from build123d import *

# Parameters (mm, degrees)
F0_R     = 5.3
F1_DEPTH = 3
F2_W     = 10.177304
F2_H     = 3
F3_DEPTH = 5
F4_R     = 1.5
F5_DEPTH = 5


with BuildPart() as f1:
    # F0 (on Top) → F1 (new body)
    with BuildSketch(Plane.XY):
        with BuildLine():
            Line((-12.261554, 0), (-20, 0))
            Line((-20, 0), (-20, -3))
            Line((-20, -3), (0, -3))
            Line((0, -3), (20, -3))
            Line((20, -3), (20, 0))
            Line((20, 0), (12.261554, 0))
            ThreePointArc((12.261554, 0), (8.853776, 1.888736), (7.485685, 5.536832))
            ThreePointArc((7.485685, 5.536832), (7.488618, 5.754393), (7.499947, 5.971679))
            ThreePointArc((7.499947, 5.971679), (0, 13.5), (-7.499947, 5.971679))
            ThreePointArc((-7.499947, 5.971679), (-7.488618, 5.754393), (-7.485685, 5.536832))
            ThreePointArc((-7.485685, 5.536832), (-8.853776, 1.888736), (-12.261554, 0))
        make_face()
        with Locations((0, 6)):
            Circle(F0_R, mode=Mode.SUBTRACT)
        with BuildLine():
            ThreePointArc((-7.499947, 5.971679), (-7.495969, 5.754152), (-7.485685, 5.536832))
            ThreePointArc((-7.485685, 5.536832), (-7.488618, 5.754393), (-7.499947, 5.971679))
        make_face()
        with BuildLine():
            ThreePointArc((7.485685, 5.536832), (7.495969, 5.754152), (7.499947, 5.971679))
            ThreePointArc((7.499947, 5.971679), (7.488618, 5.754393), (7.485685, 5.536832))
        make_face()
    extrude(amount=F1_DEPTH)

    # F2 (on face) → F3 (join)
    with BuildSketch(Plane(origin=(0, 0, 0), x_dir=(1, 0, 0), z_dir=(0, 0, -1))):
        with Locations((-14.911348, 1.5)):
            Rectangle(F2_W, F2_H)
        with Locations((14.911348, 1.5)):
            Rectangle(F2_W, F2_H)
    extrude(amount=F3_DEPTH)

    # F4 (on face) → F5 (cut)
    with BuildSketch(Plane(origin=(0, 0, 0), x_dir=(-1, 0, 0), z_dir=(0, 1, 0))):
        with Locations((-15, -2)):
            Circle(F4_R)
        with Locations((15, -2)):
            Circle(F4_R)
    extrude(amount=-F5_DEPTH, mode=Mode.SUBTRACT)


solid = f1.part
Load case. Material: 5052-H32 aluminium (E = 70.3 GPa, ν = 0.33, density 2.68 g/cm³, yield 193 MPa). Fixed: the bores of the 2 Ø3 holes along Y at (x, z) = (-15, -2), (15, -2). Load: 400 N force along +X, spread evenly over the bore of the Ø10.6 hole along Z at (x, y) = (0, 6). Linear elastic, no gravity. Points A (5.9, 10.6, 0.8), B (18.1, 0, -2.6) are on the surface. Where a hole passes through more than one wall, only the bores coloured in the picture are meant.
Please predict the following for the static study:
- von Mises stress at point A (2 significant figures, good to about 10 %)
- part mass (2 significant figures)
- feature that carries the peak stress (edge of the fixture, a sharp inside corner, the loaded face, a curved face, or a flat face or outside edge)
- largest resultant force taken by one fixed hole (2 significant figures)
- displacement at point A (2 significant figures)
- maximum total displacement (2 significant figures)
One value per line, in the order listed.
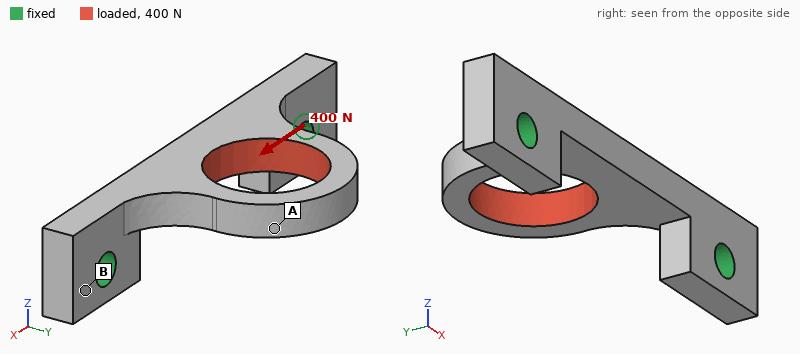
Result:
50 MPa
2.5 g
a curved face
230 N
32 µm
34 µm
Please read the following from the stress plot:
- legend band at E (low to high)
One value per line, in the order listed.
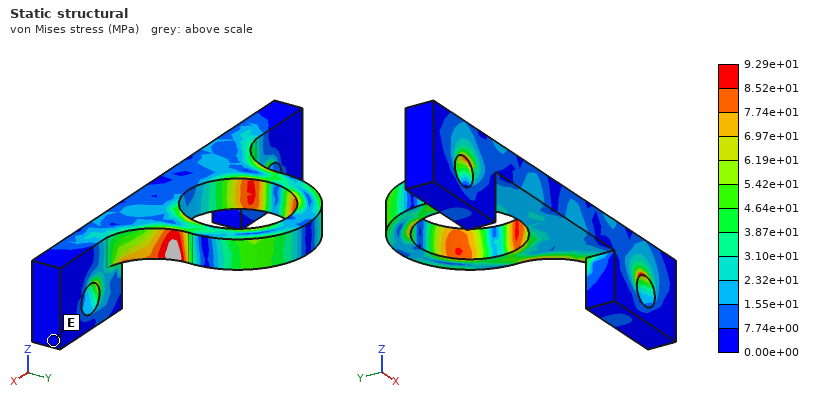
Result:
0.00e+00 to 7.74e+00 MPa
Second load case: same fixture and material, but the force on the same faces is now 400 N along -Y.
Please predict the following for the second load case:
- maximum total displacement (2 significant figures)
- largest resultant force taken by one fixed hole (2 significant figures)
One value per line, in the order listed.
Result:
34 µm
220 N
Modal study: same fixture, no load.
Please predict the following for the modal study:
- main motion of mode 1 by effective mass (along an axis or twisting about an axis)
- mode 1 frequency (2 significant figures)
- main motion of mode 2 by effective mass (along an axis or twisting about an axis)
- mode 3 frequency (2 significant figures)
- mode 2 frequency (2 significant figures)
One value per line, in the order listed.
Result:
along Z
7700 Hz
along Y
21 kHz
19 kHz
